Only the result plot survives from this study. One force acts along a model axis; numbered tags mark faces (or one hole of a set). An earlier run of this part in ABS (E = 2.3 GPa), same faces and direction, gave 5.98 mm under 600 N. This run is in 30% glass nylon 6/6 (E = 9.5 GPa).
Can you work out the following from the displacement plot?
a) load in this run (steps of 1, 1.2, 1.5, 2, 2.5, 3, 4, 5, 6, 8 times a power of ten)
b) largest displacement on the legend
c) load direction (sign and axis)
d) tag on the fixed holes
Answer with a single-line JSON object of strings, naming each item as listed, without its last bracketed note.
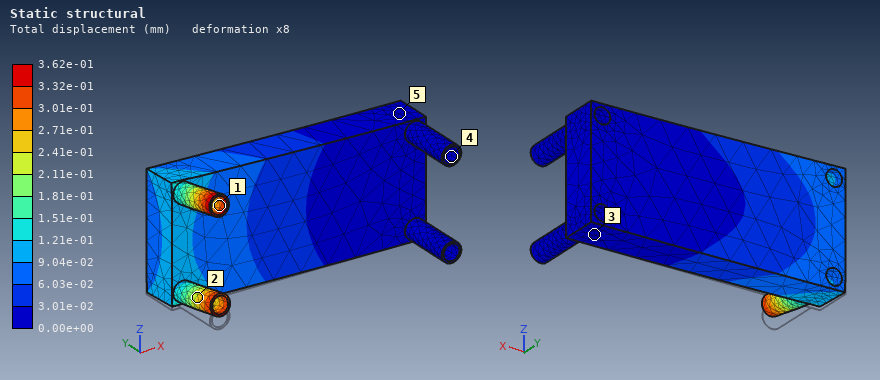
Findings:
{"load in this run": "150 N", "largest displacement on the legend": "3.62e-01 mm", "load direction": "+Z", "tag on the fixed holes": "4"}
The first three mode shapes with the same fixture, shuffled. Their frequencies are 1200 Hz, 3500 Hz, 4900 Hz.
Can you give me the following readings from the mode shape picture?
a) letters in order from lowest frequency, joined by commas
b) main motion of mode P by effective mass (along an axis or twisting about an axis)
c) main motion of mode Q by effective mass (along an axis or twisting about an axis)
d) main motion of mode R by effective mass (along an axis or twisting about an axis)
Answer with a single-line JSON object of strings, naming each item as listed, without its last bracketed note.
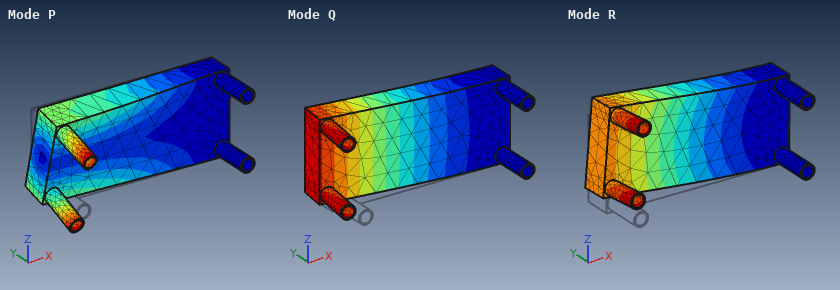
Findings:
{"letters in order from lowest frequency, joined by commas": "Q, R, P", "main motion of mode P by effective mass": "twisting about X", "main motion of mode Q by effective mass": "along Y", "main motion of mode R by effective mass": "along Z"}
